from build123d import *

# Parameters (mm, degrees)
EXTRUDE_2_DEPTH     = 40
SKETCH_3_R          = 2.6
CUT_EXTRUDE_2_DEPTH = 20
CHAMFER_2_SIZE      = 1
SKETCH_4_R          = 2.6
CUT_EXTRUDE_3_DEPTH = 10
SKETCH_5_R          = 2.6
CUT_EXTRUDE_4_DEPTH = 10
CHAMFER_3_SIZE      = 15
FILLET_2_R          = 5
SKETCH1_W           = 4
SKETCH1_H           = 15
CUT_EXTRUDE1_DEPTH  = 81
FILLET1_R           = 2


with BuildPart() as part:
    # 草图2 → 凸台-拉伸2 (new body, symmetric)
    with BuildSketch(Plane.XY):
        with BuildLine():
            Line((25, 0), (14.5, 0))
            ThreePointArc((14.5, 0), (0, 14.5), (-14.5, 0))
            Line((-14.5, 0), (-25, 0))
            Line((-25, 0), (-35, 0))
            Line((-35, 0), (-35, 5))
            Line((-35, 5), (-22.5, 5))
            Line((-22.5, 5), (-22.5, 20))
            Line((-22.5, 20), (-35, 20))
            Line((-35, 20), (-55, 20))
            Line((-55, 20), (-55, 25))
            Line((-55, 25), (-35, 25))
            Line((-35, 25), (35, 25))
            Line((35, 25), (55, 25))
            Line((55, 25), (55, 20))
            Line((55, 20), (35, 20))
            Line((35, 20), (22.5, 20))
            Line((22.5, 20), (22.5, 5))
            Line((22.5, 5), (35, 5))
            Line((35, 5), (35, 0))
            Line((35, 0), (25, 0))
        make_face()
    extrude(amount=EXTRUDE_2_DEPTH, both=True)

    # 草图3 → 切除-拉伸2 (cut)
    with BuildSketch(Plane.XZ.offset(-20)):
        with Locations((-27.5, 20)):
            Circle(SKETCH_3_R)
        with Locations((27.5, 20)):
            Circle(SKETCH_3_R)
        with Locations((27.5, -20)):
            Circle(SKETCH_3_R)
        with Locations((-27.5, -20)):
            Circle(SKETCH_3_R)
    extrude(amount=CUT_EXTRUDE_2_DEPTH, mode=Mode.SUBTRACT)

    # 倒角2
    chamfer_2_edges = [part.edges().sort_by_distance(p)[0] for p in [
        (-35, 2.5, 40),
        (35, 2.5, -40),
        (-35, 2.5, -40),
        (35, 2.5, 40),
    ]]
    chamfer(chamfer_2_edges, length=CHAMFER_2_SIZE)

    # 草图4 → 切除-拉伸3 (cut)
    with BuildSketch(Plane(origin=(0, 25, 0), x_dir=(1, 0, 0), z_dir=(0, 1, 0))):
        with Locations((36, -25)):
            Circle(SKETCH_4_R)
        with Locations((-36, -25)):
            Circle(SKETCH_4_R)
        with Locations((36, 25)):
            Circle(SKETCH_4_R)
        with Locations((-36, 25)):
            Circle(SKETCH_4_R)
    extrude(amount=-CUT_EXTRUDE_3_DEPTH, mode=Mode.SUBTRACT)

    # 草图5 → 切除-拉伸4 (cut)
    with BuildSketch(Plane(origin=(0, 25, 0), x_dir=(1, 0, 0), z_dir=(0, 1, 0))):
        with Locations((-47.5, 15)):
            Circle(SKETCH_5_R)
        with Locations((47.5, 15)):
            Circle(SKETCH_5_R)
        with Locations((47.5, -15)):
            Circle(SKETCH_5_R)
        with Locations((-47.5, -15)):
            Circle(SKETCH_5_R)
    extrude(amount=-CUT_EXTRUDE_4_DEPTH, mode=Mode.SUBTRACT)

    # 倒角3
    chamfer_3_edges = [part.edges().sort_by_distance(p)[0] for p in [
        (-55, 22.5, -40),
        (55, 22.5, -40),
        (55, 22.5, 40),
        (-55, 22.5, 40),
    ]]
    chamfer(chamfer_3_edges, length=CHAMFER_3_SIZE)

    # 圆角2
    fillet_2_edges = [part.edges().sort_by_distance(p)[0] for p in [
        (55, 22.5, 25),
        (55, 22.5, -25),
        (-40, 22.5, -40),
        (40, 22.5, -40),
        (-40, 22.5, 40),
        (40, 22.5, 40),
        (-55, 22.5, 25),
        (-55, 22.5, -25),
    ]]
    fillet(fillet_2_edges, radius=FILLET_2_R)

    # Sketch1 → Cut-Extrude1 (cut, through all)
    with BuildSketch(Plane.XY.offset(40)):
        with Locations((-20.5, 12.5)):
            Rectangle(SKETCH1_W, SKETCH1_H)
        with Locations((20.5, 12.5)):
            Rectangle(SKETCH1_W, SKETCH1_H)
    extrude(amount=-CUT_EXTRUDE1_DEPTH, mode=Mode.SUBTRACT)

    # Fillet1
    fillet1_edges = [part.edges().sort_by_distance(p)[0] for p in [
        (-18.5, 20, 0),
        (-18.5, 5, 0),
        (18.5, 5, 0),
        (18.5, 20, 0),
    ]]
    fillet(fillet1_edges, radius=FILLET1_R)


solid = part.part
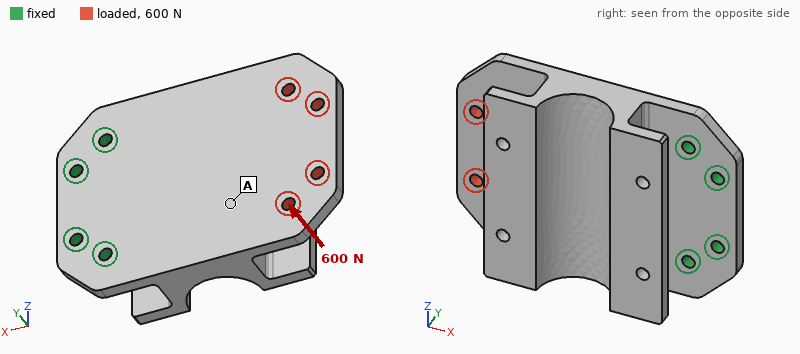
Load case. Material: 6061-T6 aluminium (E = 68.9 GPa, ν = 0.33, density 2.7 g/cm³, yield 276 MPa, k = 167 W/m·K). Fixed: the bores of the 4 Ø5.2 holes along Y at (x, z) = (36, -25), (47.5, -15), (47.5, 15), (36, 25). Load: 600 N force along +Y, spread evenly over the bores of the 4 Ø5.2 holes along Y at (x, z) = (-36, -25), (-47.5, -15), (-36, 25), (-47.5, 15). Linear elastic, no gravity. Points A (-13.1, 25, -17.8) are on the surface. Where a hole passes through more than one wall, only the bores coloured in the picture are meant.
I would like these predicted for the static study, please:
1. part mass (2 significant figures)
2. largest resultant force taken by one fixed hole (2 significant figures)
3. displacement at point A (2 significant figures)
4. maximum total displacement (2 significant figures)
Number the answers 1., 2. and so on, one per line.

1. 230 g
2. 860 N
3. 0.57 mm
4. 1.3 mm
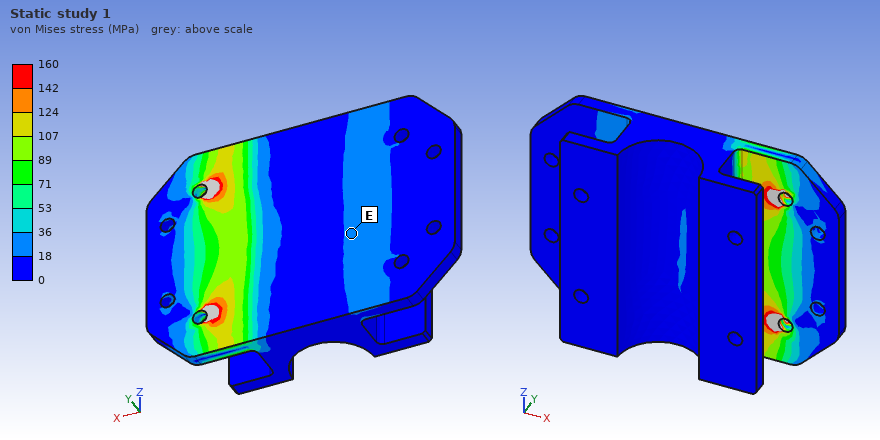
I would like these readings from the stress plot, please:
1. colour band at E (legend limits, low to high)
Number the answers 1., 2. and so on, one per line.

1. 18 to 36 MPa
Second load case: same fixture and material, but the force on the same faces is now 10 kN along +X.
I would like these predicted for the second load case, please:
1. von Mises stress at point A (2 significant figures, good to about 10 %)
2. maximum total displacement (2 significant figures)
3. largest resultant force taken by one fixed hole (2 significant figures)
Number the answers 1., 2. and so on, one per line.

1. 30 MPa
2. 0.11 mm
3. 3.4 kN
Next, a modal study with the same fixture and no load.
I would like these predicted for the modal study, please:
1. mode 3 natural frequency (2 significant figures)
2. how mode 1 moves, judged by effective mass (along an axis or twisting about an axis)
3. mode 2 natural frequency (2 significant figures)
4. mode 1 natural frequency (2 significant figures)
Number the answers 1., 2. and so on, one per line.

1. 3400 Hz
2. along Y
3. 2000 Hz
4. 470 Hz
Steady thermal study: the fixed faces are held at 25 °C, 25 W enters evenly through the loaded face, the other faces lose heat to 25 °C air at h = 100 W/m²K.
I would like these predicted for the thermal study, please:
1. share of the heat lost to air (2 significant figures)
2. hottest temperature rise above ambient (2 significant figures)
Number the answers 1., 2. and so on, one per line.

1. 61 %
2. 16 K
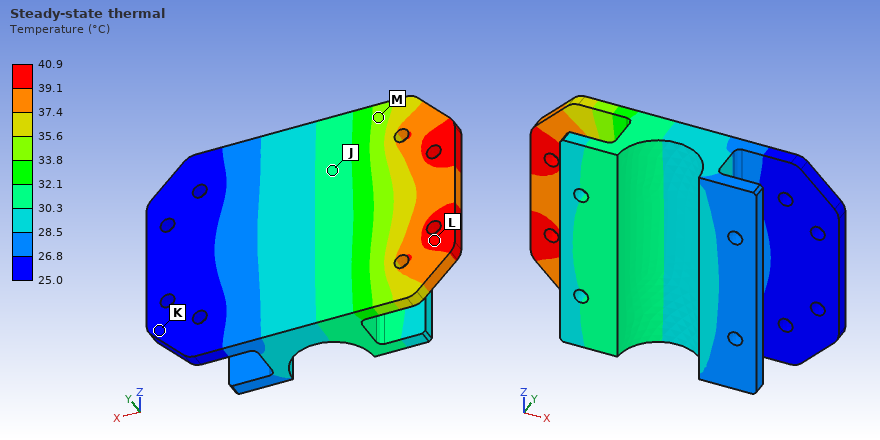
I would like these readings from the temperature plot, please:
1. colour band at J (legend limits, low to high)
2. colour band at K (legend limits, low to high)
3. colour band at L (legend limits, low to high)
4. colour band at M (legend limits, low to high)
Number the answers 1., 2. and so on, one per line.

1. 30.3 to 32.1 °C
2. 25.0 to 26.8 °C
3. 39.1 to 40.9 °C
4. 33.8 to 35.6 °C
